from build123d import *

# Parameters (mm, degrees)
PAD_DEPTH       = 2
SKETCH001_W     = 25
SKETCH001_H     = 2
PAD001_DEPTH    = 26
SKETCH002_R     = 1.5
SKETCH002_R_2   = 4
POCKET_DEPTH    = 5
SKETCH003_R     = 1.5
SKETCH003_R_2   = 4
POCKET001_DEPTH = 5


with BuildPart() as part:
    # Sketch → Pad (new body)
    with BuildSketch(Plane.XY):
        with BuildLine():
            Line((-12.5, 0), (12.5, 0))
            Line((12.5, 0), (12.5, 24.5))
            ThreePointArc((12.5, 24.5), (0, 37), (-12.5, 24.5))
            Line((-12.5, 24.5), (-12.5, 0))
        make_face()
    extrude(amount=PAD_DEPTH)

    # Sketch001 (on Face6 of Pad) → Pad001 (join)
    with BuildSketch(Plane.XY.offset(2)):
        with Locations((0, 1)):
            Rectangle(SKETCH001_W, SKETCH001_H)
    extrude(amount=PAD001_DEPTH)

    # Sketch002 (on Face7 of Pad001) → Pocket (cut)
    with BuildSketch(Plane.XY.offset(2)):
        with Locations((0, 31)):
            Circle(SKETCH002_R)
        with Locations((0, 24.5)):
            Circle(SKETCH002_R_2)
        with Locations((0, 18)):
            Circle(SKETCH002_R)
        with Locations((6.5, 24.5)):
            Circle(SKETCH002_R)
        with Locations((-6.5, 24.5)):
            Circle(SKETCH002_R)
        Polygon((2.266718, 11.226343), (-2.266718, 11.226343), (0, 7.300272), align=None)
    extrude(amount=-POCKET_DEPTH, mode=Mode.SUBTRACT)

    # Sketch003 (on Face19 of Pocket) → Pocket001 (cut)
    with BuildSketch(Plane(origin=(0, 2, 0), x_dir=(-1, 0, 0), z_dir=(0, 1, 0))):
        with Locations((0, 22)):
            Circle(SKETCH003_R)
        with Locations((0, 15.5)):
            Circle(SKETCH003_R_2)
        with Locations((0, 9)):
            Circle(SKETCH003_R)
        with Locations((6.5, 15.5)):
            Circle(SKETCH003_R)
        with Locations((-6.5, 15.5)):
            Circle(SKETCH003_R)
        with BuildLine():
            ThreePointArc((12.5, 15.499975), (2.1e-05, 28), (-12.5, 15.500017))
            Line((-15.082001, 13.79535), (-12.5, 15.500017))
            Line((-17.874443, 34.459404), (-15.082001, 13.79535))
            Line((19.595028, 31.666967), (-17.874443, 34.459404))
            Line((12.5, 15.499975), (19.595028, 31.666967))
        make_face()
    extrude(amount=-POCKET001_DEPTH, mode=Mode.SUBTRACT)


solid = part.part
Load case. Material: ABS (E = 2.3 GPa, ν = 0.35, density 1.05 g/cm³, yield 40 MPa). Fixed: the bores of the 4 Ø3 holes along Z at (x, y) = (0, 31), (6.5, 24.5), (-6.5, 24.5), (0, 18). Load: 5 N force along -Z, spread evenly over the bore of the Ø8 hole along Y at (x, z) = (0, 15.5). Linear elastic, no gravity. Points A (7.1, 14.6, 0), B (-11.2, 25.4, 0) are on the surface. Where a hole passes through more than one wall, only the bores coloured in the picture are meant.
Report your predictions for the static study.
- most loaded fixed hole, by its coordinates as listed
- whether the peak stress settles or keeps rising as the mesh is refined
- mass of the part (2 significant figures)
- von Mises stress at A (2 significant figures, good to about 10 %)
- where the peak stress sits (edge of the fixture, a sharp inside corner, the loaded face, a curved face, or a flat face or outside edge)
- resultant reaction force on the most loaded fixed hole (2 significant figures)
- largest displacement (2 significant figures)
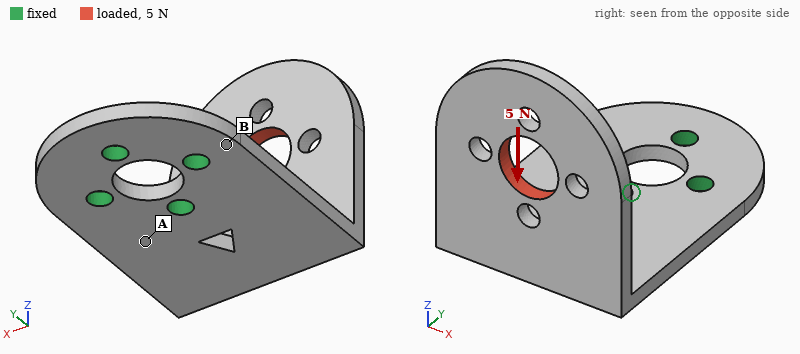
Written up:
(0, 18)
keeps rising
2.7 g
3.4 MPa
edge of the fixture
9.5 N
0.60 mm
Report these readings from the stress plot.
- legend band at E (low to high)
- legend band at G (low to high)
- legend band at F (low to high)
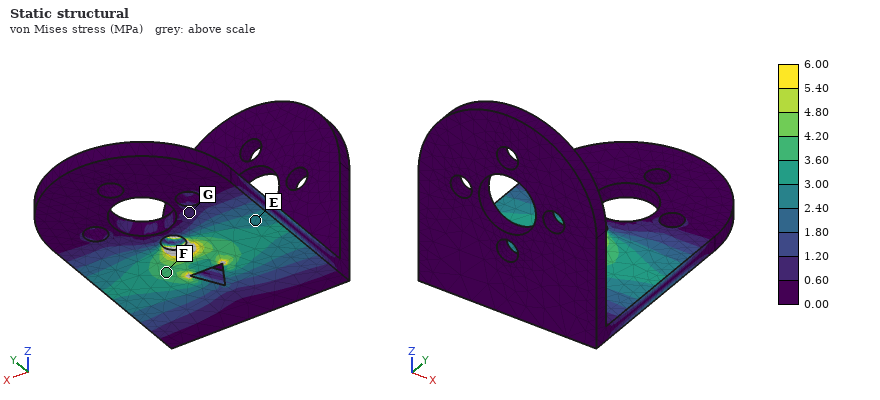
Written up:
2.40 to 3.00 MPa
0.60 to 1.20 MPa
3.60 to 4.20 MPa
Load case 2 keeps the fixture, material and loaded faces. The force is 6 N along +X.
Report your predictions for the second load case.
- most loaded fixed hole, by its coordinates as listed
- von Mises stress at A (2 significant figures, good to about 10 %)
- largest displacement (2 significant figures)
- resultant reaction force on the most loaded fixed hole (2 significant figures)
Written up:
(0, 18)
3.1 MPa
0.60 mm
7.5 N
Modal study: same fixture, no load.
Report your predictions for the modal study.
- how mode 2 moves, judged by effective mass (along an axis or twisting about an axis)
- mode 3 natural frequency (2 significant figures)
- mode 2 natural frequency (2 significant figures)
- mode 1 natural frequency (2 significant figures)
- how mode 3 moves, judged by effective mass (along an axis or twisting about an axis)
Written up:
along X
1000 Hz
570 Hz
380 Hz
along Z
